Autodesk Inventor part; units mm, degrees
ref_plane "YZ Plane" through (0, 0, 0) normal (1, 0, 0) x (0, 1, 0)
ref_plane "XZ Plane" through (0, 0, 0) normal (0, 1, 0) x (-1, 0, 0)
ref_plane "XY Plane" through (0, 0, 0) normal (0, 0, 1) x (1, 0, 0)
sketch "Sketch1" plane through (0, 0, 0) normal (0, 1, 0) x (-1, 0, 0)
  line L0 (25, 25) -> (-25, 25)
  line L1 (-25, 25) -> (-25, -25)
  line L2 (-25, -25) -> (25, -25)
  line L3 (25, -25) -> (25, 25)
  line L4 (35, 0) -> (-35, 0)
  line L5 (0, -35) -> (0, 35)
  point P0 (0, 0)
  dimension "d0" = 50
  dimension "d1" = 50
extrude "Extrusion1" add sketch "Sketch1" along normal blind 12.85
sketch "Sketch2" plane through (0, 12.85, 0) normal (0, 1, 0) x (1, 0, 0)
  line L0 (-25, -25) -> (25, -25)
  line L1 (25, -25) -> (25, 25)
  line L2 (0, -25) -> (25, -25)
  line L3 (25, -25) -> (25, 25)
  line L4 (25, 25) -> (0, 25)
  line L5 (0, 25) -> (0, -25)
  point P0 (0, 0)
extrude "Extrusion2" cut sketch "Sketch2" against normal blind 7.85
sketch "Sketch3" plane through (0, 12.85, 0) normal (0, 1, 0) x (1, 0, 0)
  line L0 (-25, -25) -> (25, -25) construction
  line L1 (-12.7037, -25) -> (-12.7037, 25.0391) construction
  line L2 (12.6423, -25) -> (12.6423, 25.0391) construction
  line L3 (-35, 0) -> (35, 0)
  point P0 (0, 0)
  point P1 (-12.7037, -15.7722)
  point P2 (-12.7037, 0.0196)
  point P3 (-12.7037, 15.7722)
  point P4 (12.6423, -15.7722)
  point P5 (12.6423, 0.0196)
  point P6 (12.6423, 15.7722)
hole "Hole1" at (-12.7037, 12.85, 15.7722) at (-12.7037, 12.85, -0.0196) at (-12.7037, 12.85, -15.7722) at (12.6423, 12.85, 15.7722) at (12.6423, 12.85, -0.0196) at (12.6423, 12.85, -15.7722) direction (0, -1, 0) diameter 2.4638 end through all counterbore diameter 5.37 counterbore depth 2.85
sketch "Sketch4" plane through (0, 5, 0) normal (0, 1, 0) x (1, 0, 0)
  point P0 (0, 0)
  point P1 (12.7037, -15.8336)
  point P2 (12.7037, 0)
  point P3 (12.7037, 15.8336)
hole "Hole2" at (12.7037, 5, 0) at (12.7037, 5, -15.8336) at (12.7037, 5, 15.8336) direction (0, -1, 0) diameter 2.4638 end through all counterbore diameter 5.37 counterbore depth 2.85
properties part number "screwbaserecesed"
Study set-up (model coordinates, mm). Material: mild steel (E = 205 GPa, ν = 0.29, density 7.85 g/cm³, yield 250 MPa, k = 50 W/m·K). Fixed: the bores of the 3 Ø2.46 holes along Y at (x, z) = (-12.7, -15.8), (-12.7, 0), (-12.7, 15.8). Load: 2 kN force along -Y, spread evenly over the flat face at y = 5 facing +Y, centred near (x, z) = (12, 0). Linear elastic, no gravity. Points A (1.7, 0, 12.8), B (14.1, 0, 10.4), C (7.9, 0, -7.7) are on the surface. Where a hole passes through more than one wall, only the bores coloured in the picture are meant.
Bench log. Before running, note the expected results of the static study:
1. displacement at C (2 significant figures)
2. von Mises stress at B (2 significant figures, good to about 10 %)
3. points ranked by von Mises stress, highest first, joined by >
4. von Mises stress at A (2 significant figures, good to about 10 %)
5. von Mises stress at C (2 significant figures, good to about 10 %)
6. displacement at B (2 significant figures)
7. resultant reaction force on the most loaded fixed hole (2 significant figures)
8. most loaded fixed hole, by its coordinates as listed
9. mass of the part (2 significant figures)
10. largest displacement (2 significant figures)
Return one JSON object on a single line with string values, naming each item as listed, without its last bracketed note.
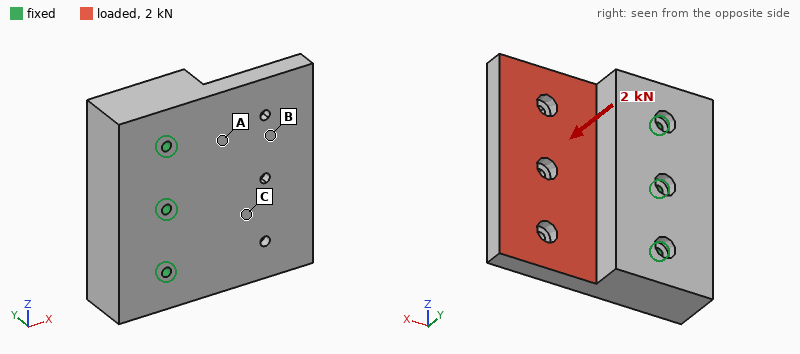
{"displacement at C": "22 µm", "von Mises stress at B": "25 MPa", "points ranked by von Mises stress, highest first, joined by >": "A > C > B", "von Mises stress at A": "90 MPa", "von Mises stress at C": "54 MPa", "displacement at B": "38 µm", "resultant reaction force on the most loaded fixed hole": "800 N", "most loaded fixed hole, by its coordinates as listed": "(-12.7, 0)", "mass of the part": "170 g", "largest displacement": "71 µm"}
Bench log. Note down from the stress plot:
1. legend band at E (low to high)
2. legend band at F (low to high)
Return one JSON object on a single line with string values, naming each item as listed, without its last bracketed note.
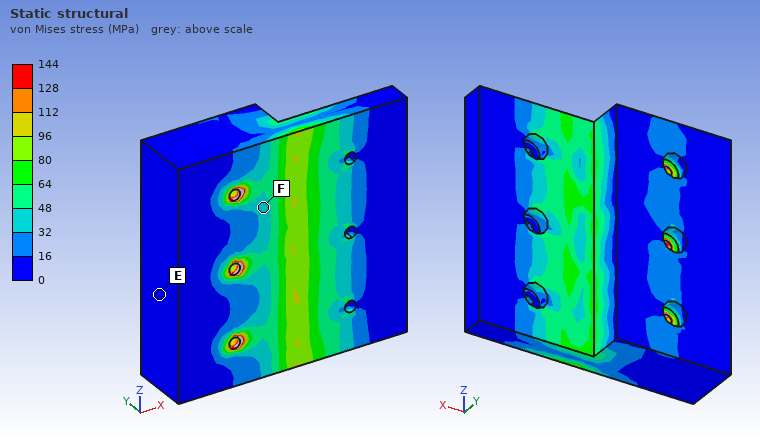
{"legend band at E": "0 to 16 MPa", "legend band at F": "32 to 48 MPa"}
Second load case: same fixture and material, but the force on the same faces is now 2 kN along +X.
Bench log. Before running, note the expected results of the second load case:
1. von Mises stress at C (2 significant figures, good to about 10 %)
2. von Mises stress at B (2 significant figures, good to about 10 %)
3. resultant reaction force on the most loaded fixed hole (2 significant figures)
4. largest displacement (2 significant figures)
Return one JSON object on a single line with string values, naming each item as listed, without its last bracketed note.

{"von Mises stress at C": "9.6 MPa", "von Mises stress at B": "8.3 MPa", "resultant reaction force on the most loaded fixed hole": "720 N", "largest displacement": "12 µm"}
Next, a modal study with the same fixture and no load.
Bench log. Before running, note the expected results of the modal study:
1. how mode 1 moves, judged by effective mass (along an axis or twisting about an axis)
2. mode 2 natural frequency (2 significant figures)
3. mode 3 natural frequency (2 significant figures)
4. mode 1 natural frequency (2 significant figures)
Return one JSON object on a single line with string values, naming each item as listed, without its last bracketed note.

{"how mode 1 moves, judged by effective mass": "along Y", "mode 2 natural frequency": "7700 Hz", "mode 3 natural frequency": "16 kHz", "mode 1 natural frequency": "4800 Hz"}
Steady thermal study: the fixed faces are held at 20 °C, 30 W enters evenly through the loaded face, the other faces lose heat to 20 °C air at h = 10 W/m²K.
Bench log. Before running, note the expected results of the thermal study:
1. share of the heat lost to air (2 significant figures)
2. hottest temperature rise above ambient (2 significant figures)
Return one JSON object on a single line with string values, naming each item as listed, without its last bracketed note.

{"share of the heat lost to air": "3.5 %", "hottest temperature rise above ambient": "50 K"}
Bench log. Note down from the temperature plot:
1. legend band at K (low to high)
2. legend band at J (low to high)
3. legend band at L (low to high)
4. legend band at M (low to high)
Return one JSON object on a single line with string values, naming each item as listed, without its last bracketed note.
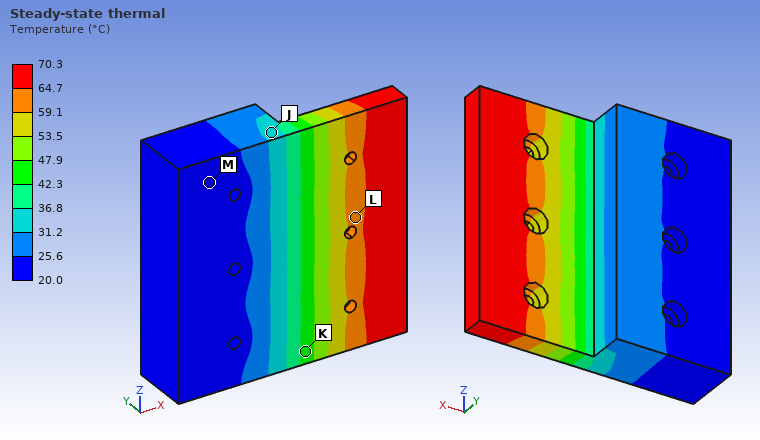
{"legend band at K": "42.3 to 47.9 °C", "legend band at J": "31.2 to 36.8 °C", "legend band at L": "59.1 to 64.7 °C", "legend band at M": "20.0 to 25.6 °C"}
